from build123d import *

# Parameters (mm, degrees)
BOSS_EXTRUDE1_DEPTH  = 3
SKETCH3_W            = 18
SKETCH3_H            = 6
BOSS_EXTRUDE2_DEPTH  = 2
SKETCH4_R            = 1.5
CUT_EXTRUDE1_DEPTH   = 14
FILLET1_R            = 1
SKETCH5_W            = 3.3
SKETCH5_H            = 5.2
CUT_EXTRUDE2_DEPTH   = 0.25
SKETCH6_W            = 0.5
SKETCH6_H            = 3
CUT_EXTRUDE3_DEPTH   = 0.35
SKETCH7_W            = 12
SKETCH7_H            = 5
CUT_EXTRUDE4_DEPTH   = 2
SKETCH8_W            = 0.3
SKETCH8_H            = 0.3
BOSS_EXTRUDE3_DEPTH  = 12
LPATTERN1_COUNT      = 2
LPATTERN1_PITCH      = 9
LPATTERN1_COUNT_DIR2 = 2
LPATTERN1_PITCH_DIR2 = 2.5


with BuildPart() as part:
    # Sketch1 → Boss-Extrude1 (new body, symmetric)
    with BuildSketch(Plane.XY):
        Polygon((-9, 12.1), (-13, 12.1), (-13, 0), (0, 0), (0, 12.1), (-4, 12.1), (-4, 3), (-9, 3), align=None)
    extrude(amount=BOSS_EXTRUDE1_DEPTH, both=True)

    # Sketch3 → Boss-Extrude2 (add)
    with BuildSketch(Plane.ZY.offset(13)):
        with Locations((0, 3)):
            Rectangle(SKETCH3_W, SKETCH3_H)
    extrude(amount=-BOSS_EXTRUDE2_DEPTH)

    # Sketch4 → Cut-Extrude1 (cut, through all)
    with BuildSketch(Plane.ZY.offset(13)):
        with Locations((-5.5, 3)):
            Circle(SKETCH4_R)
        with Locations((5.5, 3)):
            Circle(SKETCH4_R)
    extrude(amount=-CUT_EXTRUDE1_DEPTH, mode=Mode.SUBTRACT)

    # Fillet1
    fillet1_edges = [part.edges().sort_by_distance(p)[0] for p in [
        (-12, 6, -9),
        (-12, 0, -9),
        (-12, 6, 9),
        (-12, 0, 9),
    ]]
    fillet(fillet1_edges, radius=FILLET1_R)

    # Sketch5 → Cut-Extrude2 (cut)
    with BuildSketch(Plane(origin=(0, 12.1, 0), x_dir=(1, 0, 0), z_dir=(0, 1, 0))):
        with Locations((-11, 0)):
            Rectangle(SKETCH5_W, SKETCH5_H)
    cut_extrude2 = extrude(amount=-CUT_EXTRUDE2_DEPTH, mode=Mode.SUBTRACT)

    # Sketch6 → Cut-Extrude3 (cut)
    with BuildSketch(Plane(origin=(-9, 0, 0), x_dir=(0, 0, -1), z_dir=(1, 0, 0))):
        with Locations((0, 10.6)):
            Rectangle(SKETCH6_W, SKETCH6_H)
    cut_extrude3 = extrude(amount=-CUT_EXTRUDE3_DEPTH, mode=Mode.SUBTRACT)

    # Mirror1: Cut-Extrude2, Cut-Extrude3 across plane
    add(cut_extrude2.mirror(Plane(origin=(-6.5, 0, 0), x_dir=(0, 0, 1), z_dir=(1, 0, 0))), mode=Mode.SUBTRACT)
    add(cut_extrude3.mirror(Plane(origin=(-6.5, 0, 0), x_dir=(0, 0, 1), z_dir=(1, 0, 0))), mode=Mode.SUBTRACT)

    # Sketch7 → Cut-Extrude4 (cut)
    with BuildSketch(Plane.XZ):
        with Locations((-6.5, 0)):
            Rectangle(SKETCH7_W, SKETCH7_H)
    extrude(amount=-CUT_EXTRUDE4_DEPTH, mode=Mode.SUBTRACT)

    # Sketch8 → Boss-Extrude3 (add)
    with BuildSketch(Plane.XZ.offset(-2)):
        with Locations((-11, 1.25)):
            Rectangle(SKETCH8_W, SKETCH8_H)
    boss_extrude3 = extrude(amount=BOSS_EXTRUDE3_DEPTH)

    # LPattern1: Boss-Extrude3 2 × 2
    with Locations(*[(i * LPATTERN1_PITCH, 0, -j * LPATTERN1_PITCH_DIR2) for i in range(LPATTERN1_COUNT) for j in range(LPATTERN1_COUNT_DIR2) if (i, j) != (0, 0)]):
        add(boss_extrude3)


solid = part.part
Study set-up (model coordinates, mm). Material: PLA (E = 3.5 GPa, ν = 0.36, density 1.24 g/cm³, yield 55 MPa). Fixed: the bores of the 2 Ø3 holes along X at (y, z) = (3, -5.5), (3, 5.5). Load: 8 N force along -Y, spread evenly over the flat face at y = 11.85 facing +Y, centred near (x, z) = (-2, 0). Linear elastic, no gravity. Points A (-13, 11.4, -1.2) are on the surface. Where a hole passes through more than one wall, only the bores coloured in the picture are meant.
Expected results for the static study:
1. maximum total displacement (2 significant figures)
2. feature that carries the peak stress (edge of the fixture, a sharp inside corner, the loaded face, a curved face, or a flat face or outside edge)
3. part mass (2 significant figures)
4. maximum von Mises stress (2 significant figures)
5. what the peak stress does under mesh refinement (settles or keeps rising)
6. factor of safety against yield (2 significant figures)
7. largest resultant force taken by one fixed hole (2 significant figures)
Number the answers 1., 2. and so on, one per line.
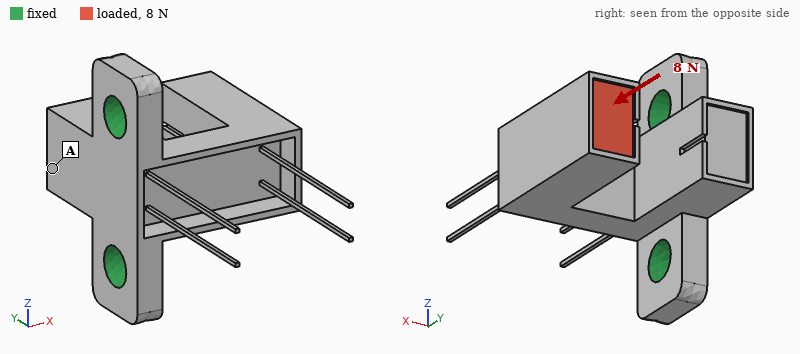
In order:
1. 0.31 mm
2. a flat face or outside edge
3. 0.82 g
4. 22 MPa
5. settles
6. 2.5
7. 4.2 N
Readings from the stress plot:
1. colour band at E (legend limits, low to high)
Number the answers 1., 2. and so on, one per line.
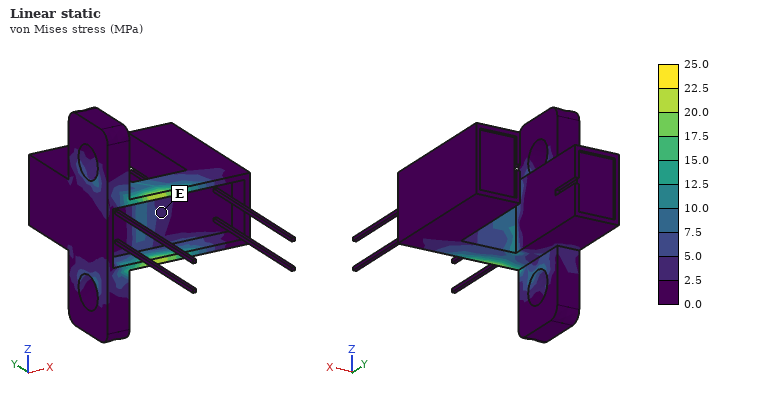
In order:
1. 2.5 to 5.0 MPa
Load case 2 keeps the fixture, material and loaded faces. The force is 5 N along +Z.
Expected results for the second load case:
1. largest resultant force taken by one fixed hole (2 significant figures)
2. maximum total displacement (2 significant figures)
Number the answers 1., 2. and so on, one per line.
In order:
1. 9.4 N
2. 0.36 mm
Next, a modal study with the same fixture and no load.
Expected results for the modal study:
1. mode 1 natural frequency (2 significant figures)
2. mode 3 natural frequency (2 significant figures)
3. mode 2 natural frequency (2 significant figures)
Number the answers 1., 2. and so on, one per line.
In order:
1. 560 Hz
2. 560 Hz
3. 560 Hz
